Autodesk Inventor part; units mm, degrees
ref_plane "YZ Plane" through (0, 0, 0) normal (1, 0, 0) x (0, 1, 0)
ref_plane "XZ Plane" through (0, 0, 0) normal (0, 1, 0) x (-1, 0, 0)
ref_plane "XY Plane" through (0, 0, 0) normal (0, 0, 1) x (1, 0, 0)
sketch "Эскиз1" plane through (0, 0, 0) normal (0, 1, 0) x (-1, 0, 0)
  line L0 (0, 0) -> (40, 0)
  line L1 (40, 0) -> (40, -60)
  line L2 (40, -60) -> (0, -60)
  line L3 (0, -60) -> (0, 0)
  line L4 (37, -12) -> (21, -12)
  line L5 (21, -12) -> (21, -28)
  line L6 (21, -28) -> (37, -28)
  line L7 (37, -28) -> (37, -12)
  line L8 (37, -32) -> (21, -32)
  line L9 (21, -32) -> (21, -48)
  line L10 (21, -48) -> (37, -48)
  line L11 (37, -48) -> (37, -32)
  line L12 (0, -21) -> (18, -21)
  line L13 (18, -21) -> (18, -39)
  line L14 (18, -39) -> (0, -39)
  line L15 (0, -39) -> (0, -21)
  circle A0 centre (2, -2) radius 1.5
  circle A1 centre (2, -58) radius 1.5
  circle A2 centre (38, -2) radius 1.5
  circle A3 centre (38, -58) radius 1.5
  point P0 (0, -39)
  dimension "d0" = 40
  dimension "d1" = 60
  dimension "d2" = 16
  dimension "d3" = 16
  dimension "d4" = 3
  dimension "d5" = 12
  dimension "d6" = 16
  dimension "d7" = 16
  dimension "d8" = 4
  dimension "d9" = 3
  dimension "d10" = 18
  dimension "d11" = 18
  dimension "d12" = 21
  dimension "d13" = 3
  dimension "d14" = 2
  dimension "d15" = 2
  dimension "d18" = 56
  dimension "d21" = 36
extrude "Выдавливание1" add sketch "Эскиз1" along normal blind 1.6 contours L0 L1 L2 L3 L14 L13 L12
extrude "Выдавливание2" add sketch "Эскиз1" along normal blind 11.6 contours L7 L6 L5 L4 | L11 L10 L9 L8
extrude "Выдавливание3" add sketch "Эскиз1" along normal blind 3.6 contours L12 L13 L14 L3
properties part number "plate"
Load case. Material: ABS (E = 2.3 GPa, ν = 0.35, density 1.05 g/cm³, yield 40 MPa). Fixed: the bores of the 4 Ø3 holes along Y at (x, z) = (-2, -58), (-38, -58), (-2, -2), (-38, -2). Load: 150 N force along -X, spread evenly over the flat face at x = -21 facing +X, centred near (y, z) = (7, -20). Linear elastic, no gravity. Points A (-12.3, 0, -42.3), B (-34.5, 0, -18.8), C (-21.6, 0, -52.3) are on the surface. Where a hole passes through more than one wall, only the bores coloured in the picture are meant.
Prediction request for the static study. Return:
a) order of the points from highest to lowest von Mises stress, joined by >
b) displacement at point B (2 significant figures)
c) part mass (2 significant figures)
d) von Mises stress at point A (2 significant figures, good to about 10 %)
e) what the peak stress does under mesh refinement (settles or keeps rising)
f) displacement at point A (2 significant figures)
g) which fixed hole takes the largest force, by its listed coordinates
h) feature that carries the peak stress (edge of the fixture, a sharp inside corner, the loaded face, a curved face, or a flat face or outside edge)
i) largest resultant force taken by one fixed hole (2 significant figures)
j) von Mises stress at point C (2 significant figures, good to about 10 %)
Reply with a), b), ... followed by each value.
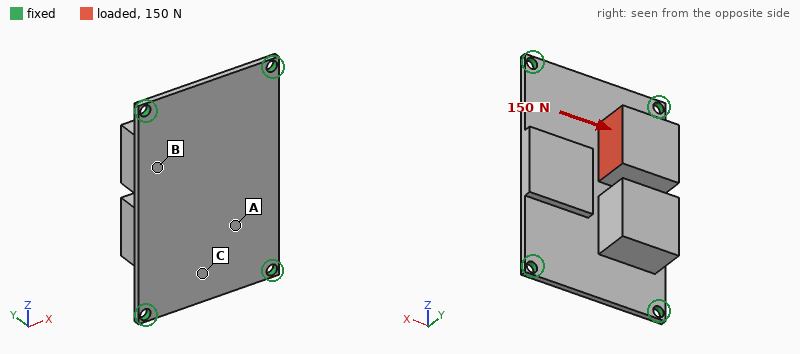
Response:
a) C > A > B
b) 0.22 mm
c) 10 g
d) 4.2 MPa
e) keeps rising
f) 0.38 mm
g) (-38, -2)
h) edge of the fixture
i) 63 N
j) 8.2 MPa
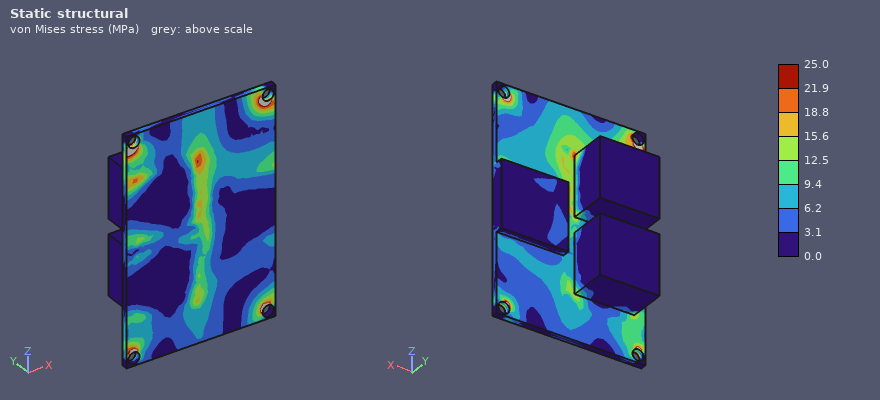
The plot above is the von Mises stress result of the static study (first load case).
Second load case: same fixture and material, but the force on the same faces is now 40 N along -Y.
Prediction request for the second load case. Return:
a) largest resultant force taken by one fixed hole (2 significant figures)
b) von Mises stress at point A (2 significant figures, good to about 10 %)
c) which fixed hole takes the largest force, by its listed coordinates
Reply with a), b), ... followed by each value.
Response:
a) 18 N
b) 4.0 MPa
c) (-38, -2)
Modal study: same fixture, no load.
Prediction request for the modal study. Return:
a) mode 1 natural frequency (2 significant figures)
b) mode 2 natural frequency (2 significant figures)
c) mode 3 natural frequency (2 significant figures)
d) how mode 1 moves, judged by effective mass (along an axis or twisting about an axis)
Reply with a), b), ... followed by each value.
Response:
a) 510 Hz
b) 880 Hz
c) 1400 Hz
d) along Y
